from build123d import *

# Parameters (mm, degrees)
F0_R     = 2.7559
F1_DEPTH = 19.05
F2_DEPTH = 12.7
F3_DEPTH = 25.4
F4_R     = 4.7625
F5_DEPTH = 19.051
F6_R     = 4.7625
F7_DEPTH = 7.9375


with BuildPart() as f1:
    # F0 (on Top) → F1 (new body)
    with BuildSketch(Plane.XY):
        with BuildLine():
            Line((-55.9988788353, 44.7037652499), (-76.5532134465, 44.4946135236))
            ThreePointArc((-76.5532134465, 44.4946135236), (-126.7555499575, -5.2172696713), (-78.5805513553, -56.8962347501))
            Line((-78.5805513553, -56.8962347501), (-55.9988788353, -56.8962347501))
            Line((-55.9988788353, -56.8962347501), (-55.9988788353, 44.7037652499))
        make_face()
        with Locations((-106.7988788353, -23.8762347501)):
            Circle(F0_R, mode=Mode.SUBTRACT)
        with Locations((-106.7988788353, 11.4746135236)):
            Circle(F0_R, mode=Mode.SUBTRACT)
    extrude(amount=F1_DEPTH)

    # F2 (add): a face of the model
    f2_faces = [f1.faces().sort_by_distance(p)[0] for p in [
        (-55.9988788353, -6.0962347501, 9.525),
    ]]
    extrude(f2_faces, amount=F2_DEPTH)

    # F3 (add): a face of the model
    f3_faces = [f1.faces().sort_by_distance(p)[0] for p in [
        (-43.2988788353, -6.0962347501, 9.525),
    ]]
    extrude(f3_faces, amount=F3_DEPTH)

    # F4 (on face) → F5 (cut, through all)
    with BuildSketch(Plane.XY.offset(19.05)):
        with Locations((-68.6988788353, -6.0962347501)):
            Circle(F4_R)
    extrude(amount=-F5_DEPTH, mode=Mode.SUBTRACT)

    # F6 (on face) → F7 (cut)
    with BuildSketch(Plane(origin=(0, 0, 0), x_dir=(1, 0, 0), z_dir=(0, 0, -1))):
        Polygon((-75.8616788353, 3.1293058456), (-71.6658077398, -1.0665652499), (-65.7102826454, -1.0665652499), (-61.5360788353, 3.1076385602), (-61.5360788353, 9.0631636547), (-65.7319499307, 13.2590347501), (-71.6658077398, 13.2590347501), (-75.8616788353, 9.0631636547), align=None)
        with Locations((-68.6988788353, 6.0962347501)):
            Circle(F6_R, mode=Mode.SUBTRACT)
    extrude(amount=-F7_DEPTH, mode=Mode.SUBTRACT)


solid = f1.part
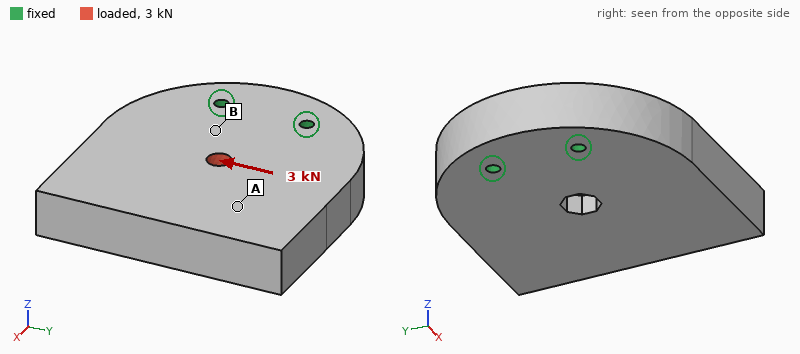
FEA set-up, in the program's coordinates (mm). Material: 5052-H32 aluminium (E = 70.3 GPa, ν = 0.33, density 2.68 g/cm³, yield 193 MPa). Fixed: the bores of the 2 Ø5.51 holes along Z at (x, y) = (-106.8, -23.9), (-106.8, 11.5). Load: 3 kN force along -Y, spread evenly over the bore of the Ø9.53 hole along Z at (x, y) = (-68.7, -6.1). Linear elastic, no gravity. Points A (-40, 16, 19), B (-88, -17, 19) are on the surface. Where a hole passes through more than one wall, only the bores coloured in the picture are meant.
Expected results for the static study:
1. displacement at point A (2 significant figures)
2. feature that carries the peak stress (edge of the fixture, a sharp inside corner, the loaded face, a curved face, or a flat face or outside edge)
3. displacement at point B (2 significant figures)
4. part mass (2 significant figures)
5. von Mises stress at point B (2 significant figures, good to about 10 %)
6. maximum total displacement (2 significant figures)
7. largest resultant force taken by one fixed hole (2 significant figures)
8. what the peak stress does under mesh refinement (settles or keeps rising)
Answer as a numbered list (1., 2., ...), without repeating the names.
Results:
1. 12 µm
2. edge of the fixture
3. 3.8 µm
4. 500 g
5. 7.6 MPa
6. 16 µm
7. 3.3 kN
8. keeps rising
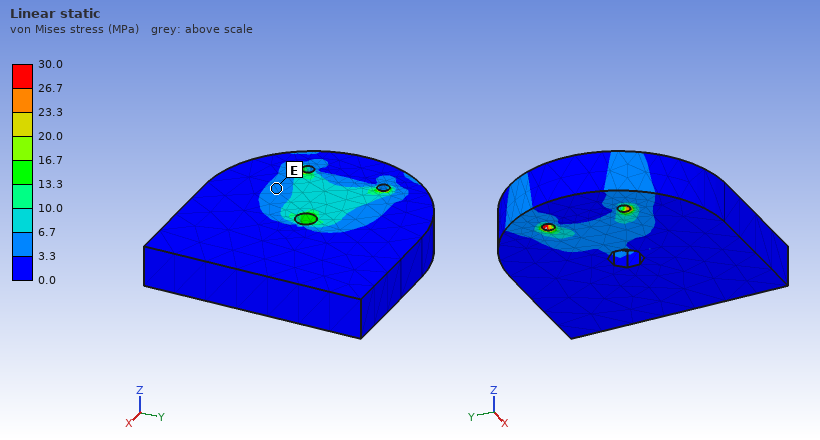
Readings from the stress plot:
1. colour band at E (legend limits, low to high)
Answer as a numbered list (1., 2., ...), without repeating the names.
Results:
1. 3.3 to 6.7 MPa
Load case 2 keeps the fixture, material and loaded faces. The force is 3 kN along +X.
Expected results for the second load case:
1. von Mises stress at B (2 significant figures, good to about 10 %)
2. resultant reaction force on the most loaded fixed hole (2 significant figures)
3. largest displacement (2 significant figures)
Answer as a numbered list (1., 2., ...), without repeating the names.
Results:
1. 5.5 MPa
2. 1.5 kN
3. 11 µm
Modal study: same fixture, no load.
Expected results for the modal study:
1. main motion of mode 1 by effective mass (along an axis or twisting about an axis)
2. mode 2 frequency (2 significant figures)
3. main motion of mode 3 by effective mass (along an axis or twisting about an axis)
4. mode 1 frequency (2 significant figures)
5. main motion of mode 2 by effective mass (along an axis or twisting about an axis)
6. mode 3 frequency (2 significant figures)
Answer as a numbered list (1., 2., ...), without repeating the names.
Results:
1. along Z
2. 3100 Hz
3. along Y
4. 1600 Hz
5. twisting about X
6. 3500 Hz
